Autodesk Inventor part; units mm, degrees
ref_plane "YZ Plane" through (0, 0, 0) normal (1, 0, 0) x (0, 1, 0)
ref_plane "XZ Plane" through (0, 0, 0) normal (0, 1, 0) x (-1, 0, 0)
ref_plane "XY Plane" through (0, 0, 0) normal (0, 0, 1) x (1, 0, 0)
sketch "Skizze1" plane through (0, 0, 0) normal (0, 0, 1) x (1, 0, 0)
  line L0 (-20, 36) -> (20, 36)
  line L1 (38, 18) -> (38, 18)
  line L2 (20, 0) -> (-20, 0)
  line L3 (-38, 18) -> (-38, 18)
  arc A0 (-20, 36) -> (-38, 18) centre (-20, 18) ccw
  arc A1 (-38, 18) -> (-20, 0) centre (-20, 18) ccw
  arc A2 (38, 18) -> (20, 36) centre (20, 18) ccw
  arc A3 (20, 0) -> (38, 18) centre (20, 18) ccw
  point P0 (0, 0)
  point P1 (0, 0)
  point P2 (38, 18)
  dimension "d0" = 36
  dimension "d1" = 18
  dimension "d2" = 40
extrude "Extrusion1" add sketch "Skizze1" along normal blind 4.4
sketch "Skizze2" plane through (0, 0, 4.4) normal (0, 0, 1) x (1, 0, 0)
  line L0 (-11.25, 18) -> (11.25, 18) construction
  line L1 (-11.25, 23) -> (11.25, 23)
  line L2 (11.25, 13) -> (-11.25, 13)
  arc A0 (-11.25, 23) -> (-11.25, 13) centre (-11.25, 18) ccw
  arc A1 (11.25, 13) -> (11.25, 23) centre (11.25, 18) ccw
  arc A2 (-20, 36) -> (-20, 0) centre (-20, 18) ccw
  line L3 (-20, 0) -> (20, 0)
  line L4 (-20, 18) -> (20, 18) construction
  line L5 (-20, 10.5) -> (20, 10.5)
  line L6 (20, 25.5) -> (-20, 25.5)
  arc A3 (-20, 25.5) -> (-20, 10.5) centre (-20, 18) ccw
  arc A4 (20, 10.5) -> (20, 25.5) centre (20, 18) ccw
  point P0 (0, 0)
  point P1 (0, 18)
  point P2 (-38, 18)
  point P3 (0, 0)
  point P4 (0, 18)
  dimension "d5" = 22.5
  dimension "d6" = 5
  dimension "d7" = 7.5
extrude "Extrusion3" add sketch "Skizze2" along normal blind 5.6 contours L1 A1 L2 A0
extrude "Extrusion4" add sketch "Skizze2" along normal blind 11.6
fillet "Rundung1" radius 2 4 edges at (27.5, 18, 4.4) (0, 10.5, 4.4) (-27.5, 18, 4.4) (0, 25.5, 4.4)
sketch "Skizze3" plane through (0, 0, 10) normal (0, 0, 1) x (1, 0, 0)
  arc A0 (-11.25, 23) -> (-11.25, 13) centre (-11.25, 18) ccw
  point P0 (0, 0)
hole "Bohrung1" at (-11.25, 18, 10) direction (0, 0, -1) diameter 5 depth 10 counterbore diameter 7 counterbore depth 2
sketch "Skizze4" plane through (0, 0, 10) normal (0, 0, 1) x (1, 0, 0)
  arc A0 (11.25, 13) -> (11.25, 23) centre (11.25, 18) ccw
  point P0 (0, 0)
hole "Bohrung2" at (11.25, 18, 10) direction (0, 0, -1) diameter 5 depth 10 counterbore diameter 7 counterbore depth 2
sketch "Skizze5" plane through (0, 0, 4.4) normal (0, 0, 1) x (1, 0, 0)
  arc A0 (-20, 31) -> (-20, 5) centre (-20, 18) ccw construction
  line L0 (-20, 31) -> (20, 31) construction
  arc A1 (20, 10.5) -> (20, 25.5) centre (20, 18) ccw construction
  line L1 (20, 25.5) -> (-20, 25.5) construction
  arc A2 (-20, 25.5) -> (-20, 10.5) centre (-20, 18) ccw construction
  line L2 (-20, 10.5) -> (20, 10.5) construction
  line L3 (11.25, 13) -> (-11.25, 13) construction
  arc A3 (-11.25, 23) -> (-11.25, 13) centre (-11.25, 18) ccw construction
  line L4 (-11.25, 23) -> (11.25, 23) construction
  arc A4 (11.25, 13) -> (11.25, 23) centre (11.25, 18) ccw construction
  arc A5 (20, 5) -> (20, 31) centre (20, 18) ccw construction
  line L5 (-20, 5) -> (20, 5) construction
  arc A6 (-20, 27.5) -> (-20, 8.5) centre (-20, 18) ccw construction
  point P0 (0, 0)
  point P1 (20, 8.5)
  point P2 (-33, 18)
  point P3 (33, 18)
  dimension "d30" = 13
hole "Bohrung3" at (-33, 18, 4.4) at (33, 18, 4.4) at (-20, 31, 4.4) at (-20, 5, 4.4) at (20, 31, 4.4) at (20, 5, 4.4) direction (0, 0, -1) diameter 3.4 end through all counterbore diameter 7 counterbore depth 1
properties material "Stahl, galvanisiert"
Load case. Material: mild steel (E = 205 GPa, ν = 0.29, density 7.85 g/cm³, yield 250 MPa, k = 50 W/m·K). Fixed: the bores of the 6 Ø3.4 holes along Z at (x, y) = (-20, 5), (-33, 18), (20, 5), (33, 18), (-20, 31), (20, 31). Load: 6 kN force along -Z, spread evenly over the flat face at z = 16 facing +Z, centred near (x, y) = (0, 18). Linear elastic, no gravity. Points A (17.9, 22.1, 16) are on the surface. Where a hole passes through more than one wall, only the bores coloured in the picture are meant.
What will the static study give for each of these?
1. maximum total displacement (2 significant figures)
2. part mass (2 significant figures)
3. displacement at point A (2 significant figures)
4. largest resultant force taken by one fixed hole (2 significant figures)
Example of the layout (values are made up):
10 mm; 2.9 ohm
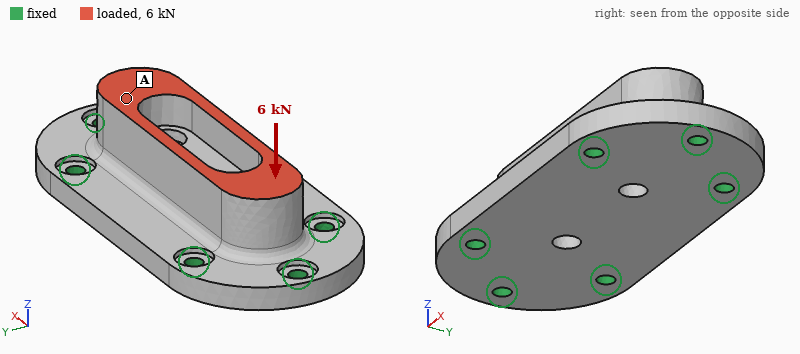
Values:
6.9 µm; 140 g; 5.0 µm; 1.3 kN
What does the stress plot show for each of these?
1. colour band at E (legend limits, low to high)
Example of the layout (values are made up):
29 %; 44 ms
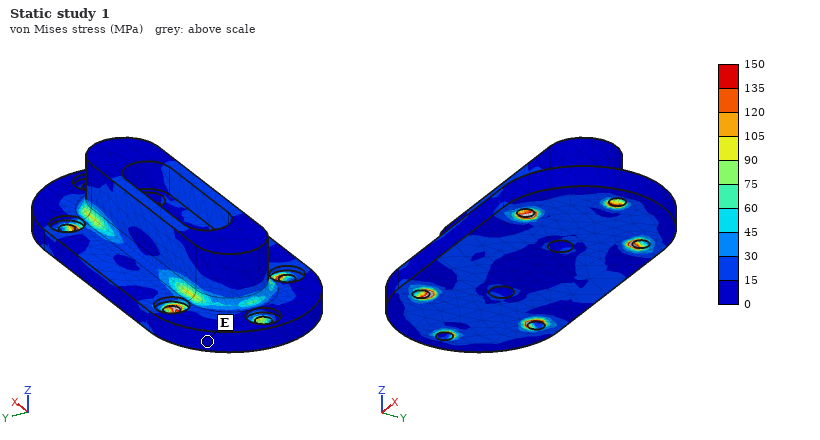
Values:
0 to 15 MPa
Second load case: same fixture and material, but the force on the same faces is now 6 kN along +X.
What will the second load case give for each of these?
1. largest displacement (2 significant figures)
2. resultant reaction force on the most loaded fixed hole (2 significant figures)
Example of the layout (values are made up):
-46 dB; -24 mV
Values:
7.2 µm; 1.4 kN
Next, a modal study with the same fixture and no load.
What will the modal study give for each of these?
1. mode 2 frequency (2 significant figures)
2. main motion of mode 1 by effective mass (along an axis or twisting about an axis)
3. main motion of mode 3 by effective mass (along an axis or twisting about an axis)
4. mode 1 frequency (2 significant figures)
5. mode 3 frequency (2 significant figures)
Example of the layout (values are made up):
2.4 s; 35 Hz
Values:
18 kHz; along Z; along Y; 14 kHz; 25 kHz
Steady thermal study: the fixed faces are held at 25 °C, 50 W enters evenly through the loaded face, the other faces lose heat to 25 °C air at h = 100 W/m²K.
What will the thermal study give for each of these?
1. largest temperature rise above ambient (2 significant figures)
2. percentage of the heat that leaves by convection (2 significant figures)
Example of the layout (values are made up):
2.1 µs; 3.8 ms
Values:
40 K; 23 %
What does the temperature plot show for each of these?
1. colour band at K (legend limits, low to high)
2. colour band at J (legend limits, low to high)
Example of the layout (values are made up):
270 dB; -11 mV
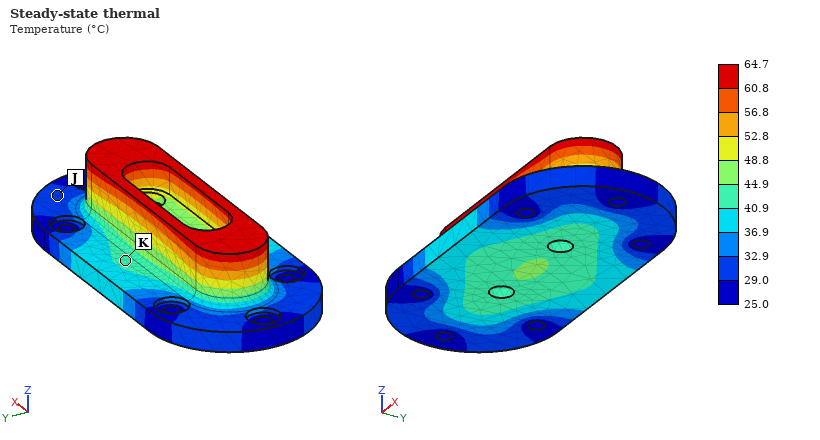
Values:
40.9 to 44.9 °C; 29.0 to 32.9 °C
